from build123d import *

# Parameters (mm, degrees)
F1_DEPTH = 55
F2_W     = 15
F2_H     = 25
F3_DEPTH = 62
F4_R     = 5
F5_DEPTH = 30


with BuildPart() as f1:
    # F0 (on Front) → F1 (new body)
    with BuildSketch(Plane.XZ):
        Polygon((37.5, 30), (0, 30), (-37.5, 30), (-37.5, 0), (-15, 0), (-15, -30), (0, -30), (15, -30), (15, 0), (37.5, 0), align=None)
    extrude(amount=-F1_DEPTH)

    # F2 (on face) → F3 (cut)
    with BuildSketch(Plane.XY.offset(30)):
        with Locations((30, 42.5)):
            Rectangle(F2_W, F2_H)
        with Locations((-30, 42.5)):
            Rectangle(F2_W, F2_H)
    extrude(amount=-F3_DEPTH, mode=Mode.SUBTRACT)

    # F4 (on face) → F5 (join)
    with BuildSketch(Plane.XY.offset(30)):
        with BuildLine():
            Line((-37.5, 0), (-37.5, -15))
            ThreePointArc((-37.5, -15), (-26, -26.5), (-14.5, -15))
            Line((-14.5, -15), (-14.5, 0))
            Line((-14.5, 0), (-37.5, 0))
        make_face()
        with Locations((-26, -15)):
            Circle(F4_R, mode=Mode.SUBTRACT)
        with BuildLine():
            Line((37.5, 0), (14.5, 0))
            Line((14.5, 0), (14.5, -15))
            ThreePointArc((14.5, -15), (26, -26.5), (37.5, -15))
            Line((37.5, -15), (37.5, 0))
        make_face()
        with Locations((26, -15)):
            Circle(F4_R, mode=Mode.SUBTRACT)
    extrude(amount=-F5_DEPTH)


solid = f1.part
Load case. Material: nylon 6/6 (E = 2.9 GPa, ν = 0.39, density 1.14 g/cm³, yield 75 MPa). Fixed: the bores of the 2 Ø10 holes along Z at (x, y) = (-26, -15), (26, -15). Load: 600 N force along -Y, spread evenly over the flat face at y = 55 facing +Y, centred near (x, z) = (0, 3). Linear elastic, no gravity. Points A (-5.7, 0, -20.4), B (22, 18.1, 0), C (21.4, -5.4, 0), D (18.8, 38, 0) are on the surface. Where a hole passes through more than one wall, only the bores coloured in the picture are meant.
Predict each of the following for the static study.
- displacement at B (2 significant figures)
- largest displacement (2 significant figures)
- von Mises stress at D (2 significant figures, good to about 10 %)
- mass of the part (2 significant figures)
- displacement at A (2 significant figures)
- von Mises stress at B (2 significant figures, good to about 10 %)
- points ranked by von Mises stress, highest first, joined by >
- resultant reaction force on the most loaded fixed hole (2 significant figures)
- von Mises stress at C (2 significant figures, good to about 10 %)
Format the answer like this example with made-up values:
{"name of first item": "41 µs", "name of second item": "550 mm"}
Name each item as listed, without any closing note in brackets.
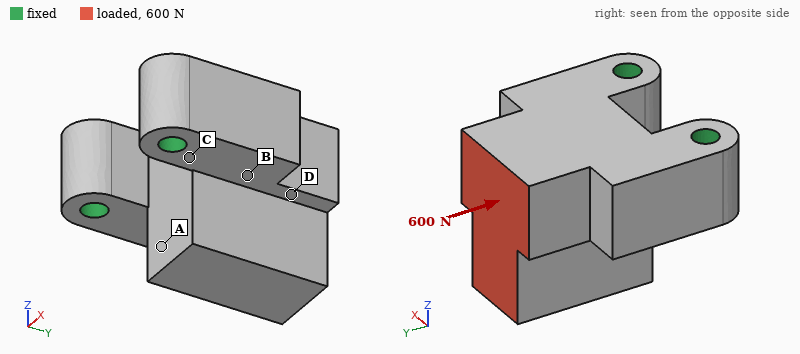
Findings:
{"displacement at B": "19 µm", "largest displacement": "70 µm", "von Mises stress at D": "0.57 MPa", "mass of the part": "200 g", "displacement at A": "39 µm", "von Mises stress at B": "1.1 MPa", "points ranked by von Mises stress, highest first, joined by >": "C > B > D > A", "resultant reaction force on the most loaded fixed hole": "310 N", "von Mises stress at C": "1.9 MPa"}
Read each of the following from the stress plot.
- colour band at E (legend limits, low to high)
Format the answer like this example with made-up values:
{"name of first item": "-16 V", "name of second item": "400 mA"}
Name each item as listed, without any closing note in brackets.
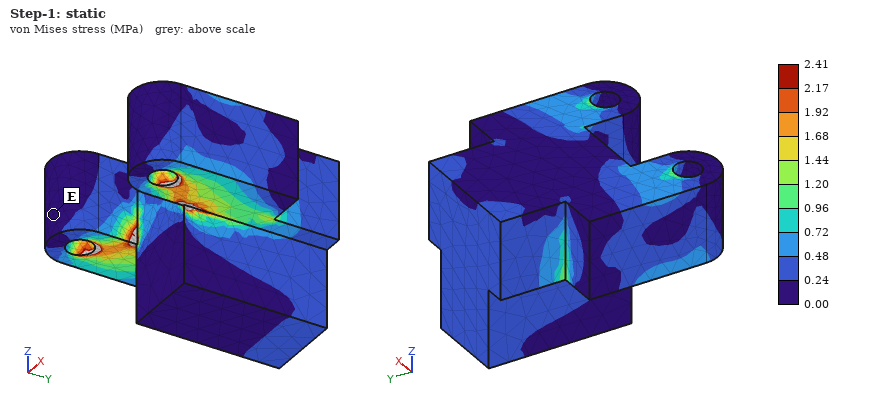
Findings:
{"colour band at E": "0.00 to 0.24 MPa"}
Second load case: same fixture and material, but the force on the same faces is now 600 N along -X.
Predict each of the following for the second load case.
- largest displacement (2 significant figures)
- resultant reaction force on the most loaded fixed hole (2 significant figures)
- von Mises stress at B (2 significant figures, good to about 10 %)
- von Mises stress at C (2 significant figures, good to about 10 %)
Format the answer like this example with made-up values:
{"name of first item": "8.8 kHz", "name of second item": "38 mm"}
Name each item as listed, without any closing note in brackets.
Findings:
{"largest displacement": "82 µm", "resultant reaction force on the most loaded fixed hole": "750 N", "von Mises stress at B": "1.4 MPa", "von Mises stress at C": "1.7 MPa"}
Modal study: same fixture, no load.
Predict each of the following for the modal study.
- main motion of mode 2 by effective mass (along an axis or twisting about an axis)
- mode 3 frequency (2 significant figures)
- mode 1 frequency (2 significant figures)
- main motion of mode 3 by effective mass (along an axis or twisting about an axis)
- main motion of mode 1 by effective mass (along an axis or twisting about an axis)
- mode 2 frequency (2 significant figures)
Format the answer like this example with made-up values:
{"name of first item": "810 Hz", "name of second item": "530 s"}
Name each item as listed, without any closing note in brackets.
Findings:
{"main motion of mode 2 by effective mass": "along X", "mode 3 frequency": "2700 Hz", "mode 1 frequency": "990 Hz", "main motion of mode 3 by effective mass": "along X", "main motion of mode 1 by effective mass": "along Z", "mode 2 frequency": "1800 Hz"}
